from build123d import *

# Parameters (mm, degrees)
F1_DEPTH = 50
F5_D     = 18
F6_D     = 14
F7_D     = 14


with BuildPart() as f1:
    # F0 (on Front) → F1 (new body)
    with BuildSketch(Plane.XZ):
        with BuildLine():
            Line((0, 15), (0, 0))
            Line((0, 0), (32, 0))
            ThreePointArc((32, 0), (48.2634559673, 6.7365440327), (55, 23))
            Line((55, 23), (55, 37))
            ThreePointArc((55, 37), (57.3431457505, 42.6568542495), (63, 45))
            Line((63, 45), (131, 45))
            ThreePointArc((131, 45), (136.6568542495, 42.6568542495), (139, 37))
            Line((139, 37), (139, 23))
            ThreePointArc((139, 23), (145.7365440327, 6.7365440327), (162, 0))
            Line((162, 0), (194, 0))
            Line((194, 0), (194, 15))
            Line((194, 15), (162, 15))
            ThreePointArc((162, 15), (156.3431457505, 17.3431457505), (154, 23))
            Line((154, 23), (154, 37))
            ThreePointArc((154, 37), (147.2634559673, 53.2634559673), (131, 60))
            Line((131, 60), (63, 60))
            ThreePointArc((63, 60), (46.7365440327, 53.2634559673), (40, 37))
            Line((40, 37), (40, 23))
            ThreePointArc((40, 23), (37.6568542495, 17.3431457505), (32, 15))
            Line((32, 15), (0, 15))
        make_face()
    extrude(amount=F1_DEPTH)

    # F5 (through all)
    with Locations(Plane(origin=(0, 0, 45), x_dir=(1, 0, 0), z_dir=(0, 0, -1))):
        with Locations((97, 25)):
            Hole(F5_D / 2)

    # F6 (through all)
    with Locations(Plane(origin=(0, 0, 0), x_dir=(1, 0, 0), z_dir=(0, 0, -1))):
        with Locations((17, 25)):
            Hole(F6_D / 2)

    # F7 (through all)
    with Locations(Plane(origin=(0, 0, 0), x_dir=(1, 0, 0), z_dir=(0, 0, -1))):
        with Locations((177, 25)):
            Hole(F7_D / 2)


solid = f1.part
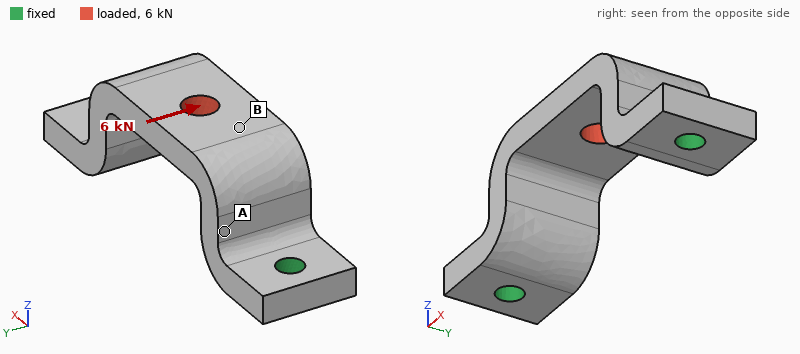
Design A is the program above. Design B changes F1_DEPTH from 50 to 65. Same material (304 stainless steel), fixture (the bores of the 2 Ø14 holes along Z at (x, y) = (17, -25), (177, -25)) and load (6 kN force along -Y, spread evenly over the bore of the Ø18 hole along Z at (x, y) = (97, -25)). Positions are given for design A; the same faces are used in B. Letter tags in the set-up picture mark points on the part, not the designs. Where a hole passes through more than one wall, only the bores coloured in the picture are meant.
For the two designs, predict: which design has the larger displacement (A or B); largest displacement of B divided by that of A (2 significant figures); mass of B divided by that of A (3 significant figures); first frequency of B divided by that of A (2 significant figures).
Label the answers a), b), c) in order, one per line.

a) A
b) 0.91
c) 1.31
d) 0.89
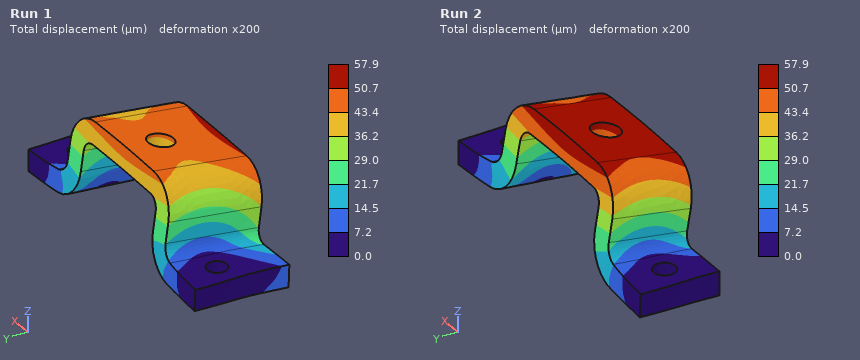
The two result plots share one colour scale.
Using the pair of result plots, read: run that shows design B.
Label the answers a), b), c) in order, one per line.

a) Run 1
